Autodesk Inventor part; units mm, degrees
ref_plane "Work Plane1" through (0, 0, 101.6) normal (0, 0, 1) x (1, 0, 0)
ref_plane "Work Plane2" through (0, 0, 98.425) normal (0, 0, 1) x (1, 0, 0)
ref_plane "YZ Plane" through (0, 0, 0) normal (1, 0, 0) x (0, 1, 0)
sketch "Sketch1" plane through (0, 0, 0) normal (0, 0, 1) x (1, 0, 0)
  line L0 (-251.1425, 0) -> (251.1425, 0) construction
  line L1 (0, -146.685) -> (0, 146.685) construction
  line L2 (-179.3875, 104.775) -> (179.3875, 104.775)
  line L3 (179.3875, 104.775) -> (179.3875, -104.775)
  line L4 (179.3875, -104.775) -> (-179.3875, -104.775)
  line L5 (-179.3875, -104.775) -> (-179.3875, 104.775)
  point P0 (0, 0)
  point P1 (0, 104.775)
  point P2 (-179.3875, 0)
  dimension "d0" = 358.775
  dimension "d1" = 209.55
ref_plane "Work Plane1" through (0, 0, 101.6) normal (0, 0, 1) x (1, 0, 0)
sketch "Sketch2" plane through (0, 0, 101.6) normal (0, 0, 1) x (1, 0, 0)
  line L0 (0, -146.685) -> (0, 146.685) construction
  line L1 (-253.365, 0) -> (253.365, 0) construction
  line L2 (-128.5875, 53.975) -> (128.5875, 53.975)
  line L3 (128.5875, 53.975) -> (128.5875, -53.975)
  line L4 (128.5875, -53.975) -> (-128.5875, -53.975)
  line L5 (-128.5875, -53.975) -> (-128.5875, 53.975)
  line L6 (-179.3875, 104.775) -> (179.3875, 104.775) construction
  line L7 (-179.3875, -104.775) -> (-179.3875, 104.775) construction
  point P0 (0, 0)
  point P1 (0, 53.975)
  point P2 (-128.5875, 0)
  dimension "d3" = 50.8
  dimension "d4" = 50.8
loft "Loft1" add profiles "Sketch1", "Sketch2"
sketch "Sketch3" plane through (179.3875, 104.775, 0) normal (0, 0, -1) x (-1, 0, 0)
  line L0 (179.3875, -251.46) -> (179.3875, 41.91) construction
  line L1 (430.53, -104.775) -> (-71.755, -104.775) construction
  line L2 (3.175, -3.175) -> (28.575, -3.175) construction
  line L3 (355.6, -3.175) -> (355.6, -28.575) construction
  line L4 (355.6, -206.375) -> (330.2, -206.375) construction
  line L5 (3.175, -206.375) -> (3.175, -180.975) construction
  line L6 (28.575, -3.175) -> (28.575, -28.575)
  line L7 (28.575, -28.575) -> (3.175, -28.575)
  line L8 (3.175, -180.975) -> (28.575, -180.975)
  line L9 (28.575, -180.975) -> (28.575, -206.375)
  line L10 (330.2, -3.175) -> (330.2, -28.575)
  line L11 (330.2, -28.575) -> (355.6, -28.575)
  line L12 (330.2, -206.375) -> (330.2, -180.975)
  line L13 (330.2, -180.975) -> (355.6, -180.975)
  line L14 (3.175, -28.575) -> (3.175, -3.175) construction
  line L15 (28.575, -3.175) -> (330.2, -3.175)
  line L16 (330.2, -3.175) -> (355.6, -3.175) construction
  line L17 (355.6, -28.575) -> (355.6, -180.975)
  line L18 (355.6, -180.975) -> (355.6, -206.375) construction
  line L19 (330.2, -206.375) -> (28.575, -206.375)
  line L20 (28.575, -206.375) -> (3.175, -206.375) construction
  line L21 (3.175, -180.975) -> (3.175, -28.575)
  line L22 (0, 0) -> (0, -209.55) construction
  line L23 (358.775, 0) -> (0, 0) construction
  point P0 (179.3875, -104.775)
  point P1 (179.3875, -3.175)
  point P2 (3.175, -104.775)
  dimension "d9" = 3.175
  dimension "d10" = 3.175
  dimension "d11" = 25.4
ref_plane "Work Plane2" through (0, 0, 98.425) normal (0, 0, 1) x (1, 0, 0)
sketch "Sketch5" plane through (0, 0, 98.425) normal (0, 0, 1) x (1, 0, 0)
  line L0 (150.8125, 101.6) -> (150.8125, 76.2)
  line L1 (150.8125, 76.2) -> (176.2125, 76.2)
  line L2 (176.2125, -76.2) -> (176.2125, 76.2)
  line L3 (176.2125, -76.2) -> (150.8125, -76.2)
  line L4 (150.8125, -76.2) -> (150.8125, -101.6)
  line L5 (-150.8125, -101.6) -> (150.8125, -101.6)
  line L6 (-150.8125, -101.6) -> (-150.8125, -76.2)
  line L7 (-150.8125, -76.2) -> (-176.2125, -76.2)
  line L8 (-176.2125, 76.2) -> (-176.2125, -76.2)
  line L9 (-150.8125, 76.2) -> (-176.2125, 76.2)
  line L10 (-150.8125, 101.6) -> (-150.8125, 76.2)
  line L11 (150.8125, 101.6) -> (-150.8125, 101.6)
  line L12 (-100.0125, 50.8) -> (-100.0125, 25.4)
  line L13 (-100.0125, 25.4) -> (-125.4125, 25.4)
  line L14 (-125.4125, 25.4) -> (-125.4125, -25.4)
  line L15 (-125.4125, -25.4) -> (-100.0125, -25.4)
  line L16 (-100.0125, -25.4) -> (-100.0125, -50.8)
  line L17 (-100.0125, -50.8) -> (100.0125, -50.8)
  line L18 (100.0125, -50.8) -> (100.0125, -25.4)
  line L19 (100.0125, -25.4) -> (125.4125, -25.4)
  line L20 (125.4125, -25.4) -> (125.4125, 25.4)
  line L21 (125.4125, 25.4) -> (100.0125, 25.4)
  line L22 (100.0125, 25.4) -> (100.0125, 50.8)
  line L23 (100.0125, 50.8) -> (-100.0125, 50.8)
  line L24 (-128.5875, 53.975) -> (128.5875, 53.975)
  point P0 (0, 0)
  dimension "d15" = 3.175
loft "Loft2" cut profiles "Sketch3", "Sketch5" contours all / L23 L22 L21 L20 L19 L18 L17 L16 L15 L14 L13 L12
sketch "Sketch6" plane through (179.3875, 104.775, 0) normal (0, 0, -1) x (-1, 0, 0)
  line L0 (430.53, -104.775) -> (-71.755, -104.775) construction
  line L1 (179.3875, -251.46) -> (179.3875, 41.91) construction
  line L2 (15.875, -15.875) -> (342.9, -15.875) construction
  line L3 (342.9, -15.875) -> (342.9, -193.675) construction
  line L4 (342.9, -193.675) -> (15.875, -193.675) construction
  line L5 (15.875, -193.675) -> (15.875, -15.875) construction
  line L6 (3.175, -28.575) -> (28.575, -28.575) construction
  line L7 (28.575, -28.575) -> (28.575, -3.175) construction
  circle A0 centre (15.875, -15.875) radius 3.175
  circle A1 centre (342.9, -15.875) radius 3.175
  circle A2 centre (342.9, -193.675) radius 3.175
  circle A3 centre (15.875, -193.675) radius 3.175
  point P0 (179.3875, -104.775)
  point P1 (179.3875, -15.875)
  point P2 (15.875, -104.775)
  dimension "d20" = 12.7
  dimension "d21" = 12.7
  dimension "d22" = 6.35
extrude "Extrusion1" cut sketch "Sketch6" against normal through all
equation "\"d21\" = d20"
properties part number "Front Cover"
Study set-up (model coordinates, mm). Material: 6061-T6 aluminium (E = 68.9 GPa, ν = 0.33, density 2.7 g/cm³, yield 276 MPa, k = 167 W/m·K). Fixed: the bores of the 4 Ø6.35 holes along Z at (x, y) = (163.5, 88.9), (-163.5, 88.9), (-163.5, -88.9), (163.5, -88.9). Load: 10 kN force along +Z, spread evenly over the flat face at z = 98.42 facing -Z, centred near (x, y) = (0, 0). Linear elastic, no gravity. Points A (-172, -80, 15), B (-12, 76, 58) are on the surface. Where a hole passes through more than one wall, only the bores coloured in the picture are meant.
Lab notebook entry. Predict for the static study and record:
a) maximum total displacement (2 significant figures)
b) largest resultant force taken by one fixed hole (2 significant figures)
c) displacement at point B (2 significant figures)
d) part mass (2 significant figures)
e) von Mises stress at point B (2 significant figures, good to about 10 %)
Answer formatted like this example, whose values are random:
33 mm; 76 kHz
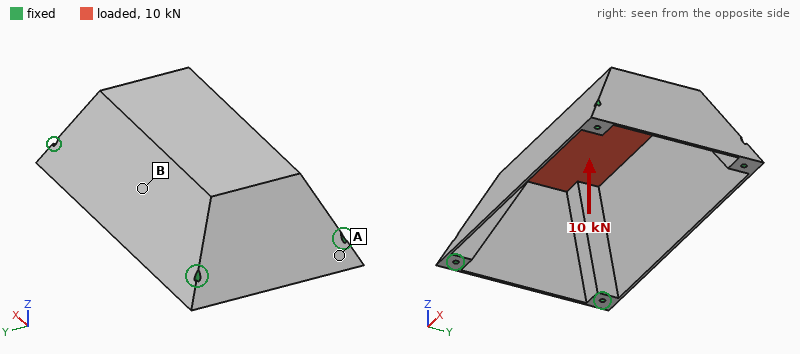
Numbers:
1.2 mm; 3.6 kN; 0.74 mm; 1.9 kg; 30 MPa
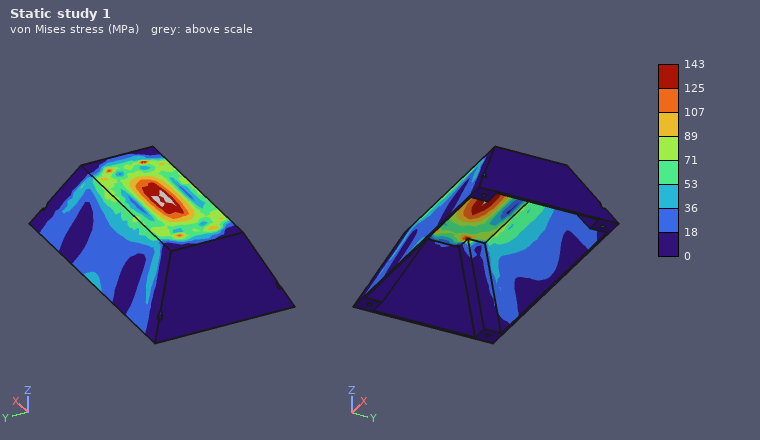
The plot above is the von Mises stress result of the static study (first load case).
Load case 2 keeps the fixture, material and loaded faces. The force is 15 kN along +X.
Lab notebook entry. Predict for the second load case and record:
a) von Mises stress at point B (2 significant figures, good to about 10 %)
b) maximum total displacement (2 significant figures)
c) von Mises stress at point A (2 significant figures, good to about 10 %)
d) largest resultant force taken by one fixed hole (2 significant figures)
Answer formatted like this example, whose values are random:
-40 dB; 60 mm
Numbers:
10 MPa; 46 µm; 8.0 MPa; 4.2 kN
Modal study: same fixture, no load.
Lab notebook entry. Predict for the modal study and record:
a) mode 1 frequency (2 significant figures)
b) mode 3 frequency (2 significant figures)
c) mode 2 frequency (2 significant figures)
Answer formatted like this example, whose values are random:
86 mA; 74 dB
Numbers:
370 Hz; 790 Hz; 390 Hz
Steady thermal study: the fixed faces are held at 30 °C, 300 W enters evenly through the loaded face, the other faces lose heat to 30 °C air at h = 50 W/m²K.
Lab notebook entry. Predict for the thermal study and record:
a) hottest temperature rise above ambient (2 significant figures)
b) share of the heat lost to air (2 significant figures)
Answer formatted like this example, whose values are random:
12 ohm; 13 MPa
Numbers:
62 K; 67 %
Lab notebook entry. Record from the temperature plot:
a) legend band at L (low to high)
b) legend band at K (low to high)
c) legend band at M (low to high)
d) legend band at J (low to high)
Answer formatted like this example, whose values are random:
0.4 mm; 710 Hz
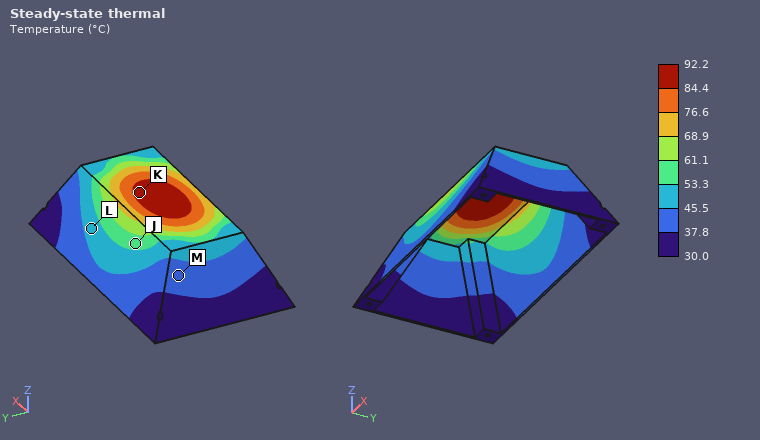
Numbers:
45.5 to 53.3 °C; 84.4 to 92.2 °C; 37.8 to 45.5 °C; 53.3 to 61.1 °C
